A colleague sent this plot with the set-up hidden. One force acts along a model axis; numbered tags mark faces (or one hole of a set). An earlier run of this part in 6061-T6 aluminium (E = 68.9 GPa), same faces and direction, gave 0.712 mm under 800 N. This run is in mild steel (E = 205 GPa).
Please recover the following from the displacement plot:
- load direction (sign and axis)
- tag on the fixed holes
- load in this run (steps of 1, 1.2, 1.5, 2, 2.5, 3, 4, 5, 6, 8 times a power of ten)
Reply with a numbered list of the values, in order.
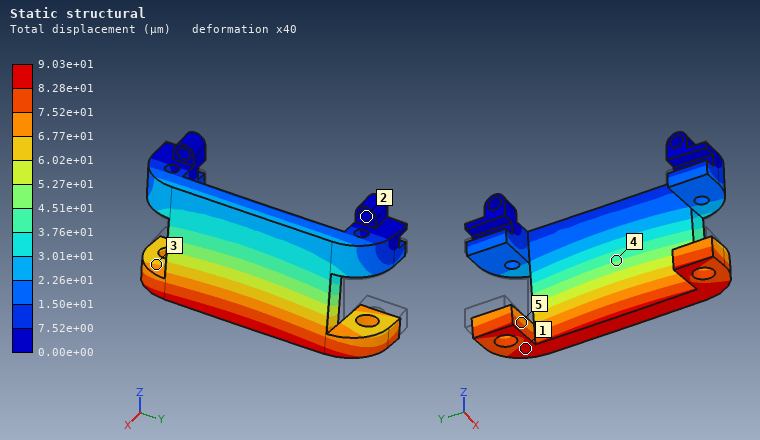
1. +X
2. 2
3. 300 N
